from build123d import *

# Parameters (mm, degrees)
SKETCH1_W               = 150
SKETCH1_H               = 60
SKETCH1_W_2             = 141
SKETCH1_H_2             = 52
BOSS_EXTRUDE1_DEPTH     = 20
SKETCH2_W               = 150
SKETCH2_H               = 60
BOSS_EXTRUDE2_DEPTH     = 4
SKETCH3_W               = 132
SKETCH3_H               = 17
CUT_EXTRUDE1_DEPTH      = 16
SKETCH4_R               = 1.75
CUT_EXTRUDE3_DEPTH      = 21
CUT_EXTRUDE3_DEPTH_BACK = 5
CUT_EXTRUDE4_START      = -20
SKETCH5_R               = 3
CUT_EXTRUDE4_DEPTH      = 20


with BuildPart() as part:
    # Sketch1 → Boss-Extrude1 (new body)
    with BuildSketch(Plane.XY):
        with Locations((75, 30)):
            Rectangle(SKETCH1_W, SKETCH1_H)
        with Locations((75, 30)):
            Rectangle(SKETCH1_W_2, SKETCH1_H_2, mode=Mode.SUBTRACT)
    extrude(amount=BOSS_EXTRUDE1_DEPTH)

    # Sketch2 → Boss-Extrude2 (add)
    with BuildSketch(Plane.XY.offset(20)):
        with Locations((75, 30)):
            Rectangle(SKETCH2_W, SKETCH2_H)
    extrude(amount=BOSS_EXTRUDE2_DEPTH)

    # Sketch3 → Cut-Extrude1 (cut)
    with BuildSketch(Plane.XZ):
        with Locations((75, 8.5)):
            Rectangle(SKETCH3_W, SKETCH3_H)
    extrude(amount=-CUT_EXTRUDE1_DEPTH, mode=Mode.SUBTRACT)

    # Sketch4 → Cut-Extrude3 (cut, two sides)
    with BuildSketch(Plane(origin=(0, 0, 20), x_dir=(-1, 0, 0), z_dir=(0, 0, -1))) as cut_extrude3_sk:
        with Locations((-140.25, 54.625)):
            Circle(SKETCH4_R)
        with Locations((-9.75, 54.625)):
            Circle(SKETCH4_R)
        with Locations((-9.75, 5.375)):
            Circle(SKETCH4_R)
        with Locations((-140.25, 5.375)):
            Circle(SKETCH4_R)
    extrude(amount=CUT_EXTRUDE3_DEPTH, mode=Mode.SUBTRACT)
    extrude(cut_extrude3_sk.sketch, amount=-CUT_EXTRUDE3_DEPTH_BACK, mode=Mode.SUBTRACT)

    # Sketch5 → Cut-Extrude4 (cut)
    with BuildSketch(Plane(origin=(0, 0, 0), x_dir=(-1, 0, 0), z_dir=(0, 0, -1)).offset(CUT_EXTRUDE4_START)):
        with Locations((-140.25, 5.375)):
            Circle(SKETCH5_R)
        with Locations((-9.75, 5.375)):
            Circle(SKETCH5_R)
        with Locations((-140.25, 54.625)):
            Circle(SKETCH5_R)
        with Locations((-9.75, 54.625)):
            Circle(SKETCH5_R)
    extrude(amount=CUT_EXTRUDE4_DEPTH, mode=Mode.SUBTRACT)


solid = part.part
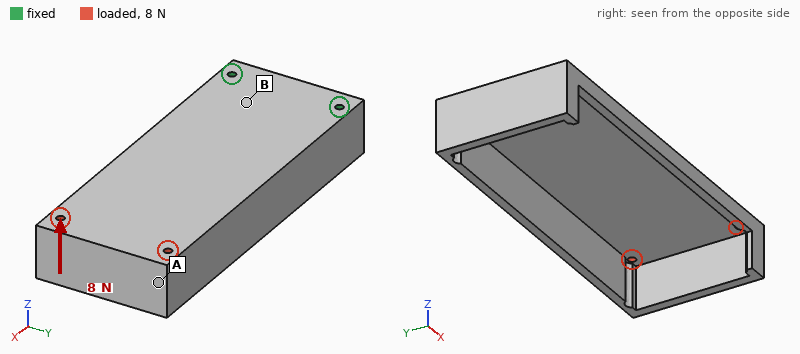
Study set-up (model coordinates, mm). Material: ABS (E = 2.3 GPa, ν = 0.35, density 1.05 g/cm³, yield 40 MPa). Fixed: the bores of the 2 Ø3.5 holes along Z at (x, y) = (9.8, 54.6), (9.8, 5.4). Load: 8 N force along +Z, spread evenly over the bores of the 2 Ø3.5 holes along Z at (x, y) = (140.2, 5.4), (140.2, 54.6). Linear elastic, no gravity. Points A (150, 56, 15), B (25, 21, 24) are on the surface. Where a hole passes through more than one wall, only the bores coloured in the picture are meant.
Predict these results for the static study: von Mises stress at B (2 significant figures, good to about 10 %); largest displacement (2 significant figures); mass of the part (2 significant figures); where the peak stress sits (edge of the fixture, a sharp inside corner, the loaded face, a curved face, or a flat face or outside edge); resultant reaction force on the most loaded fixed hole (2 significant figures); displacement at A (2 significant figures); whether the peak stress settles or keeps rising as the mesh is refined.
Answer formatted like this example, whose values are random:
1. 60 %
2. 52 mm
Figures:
1. 1.00 MPa
2. 1.9 mm
3. 63 g
4. edge of the fixture
5. 5.8 N
6. 1.4 mm
7. keeps rising
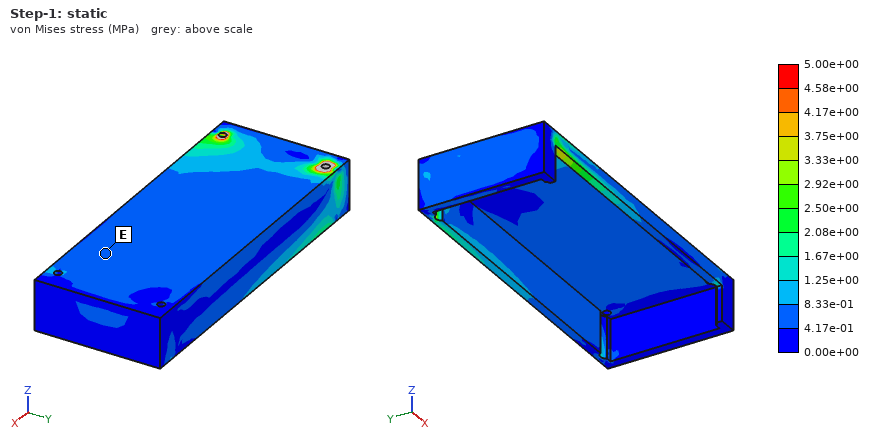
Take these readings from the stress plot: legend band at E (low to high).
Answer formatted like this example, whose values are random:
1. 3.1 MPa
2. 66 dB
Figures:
1. 4.17e-01 to 8.33e-01 MPa
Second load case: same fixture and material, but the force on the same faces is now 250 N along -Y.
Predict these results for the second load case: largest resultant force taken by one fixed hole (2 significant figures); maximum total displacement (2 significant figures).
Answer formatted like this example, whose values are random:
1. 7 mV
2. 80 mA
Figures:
1. 660 N
2. 1.8 mm
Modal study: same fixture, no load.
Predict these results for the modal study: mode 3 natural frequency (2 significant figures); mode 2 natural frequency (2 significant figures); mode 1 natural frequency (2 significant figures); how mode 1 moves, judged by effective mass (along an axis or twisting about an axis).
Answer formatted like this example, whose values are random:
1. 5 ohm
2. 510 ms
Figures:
1. 490 Hz
2. 190 Hz
3. 77 Hz
4. along Z
